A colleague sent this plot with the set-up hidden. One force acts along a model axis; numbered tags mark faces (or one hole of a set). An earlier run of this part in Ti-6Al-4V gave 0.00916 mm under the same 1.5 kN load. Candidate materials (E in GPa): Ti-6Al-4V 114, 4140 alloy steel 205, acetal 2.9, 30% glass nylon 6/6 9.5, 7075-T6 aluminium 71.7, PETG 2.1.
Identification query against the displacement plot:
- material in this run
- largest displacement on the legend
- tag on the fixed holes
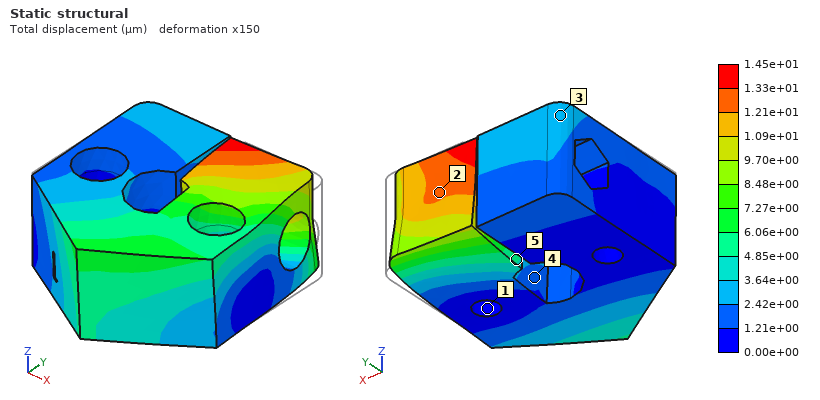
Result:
7075-T6 aluminium
1.45e+01 µm
1
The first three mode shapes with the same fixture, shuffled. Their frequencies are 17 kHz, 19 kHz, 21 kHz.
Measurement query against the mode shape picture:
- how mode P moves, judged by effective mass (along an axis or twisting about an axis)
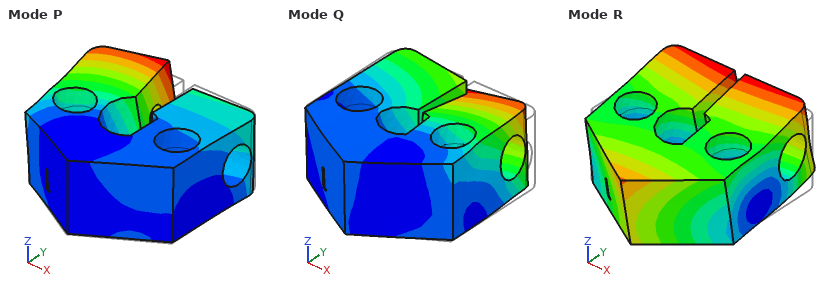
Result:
along X
